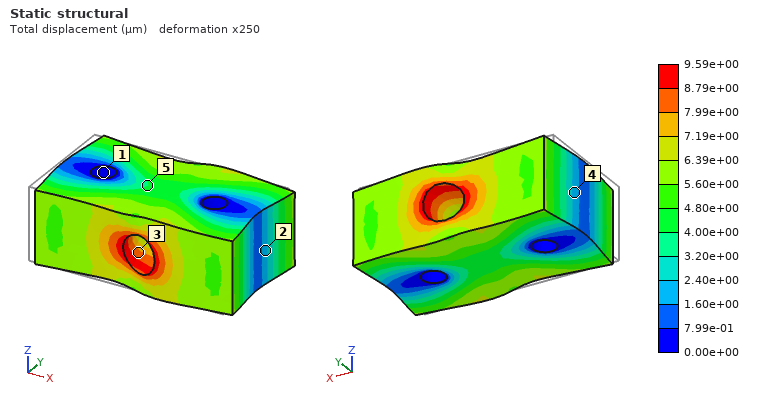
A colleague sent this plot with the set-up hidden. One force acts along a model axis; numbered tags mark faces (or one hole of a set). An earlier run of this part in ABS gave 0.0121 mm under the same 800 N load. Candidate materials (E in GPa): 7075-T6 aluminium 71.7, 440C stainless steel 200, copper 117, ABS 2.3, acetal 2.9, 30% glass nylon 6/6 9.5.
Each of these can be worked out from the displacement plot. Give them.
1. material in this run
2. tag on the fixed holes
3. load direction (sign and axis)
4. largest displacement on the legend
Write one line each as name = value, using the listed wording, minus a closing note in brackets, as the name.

material in this run = acetal
tag on the fixed holes = 1
load direction = +X
largest displacement on the legend = 9.59e+00 µm
